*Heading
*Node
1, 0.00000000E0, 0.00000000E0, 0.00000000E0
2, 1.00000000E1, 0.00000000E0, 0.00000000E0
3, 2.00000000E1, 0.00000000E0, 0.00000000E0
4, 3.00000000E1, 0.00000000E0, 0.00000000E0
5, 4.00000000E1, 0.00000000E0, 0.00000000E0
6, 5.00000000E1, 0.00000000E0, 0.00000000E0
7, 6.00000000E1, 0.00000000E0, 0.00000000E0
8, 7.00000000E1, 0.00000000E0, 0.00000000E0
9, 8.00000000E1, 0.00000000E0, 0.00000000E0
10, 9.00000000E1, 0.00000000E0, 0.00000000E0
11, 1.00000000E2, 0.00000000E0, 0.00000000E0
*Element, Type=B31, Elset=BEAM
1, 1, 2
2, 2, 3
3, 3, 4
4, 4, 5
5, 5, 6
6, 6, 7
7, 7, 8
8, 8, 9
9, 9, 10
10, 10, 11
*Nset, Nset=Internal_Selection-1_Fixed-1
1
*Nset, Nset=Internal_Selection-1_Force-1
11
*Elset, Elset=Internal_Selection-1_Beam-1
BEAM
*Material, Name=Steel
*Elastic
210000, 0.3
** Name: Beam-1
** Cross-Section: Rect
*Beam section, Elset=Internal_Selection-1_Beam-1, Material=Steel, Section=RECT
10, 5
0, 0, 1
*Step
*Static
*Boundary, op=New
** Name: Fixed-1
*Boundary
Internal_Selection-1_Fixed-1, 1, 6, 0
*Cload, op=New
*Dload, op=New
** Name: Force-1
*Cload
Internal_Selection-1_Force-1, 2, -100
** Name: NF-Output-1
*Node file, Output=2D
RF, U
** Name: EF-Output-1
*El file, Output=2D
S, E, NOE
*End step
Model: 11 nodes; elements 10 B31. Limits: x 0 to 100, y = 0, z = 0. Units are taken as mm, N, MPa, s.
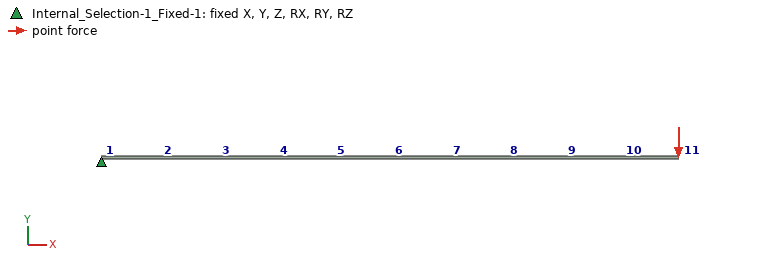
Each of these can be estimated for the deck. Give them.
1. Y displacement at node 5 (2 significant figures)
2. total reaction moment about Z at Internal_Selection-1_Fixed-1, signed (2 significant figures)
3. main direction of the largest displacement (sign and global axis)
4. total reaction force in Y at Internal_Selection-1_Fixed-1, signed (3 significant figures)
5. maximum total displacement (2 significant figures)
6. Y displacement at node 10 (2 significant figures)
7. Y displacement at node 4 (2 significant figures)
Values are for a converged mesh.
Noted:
-0.32 mm
10000 N·mm
-Y
100 N
1.5 mm
-1.3 mm
-0.19 mm
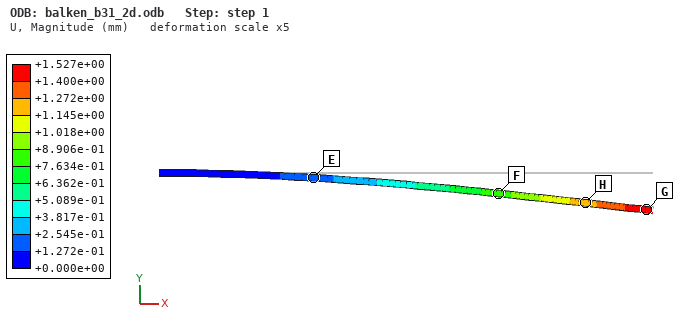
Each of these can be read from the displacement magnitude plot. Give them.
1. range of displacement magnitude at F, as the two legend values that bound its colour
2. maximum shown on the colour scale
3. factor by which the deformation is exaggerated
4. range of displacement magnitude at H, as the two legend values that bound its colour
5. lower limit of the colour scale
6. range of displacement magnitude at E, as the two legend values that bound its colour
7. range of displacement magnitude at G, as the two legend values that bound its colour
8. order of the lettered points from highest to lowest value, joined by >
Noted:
+7.634e-01 to +8.906e-01 mm
+1.527e+00 mm
5
+1.145e+00 to +1.272e+00 mm
+0.000e+00 mm
+1.272e-01 to +2.545e-01 mm
+1.400e+00 to +1.527e+00 mm
G > H > F > E
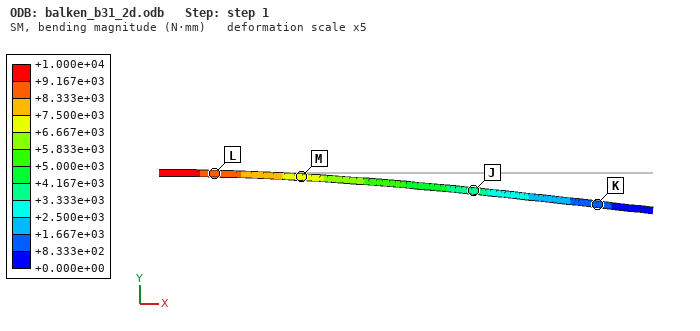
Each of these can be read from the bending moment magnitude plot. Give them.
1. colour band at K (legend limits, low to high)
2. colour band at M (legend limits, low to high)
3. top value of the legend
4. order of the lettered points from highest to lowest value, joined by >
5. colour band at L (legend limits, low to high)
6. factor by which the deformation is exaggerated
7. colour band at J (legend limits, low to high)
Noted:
+8.333e+02 to +1.667e+03 N·mm
+6.667e+03 to +7.500e+03 N·mm
+1.000e+04 N·mm
L > M > J > K
+8.333e+03 to +9.167e+03 N·mm
5
+3.333e+03 to +4.167e+03 N·mm
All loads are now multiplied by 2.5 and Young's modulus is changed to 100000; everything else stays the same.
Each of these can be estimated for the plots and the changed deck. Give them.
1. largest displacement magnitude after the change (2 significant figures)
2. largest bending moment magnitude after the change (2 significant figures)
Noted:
8.0 mm
25000 N·mm
